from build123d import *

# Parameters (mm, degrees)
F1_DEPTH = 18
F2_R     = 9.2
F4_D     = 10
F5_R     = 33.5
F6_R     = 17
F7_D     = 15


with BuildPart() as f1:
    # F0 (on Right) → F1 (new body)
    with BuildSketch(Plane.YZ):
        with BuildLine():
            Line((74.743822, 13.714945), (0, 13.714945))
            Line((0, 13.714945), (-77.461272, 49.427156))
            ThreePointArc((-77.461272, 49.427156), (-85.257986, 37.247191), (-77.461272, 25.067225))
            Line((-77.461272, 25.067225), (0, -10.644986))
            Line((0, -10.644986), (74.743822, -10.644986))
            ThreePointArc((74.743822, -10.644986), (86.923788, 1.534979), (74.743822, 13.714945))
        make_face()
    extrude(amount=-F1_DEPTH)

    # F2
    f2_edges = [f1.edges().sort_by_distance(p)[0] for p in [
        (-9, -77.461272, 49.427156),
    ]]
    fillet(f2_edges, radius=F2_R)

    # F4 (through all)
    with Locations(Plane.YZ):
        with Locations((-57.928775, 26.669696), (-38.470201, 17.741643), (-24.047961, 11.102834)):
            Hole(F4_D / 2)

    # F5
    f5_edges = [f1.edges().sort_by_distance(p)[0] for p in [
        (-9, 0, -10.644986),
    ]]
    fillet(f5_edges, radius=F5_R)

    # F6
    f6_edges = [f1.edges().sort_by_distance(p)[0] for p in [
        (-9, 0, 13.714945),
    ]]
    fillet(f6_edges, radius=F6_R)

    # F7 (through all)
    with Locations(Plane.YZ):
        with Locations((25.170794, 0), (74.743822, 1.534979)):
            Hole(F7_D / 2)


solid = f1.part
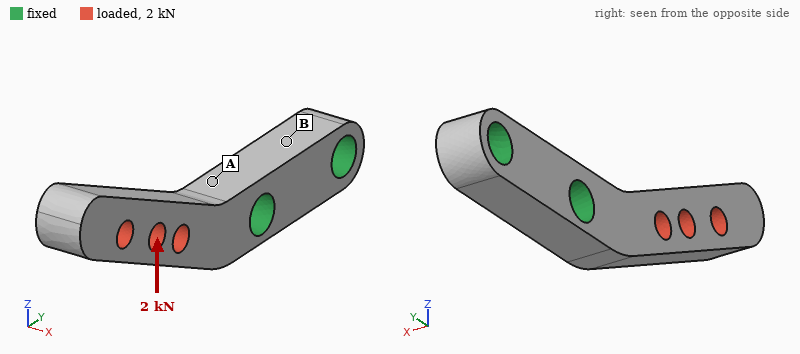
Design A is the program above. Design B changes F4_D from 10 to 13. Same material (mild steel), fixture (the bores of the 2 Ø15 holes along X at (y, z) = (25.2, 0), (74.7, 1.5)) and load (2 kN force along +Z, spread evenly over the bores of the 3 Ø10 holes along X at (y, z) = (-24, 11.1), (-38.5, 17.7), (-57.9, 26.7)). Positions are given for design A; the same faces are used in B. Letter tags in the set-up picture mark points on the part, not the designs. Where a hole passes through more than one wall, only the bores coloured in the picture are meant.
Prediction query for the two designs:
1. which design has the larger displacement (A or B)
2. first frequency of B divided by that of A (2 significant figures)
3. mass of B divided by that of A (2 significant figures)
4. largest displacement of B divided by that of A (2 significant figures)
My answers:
B
0.98
0.95
1.1
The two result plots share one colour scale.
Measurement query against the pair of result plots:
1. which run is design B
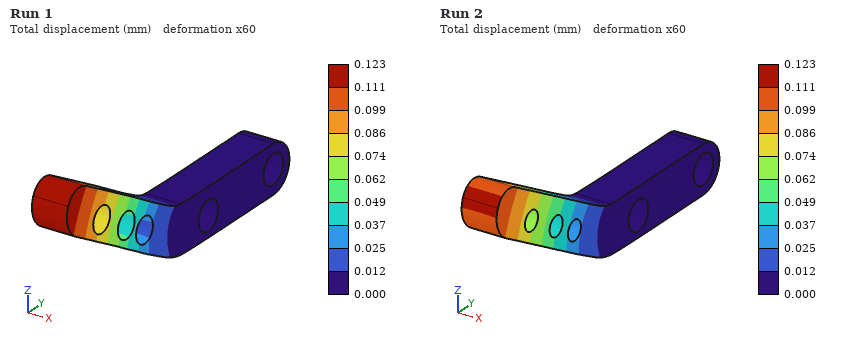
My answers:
Run 1
